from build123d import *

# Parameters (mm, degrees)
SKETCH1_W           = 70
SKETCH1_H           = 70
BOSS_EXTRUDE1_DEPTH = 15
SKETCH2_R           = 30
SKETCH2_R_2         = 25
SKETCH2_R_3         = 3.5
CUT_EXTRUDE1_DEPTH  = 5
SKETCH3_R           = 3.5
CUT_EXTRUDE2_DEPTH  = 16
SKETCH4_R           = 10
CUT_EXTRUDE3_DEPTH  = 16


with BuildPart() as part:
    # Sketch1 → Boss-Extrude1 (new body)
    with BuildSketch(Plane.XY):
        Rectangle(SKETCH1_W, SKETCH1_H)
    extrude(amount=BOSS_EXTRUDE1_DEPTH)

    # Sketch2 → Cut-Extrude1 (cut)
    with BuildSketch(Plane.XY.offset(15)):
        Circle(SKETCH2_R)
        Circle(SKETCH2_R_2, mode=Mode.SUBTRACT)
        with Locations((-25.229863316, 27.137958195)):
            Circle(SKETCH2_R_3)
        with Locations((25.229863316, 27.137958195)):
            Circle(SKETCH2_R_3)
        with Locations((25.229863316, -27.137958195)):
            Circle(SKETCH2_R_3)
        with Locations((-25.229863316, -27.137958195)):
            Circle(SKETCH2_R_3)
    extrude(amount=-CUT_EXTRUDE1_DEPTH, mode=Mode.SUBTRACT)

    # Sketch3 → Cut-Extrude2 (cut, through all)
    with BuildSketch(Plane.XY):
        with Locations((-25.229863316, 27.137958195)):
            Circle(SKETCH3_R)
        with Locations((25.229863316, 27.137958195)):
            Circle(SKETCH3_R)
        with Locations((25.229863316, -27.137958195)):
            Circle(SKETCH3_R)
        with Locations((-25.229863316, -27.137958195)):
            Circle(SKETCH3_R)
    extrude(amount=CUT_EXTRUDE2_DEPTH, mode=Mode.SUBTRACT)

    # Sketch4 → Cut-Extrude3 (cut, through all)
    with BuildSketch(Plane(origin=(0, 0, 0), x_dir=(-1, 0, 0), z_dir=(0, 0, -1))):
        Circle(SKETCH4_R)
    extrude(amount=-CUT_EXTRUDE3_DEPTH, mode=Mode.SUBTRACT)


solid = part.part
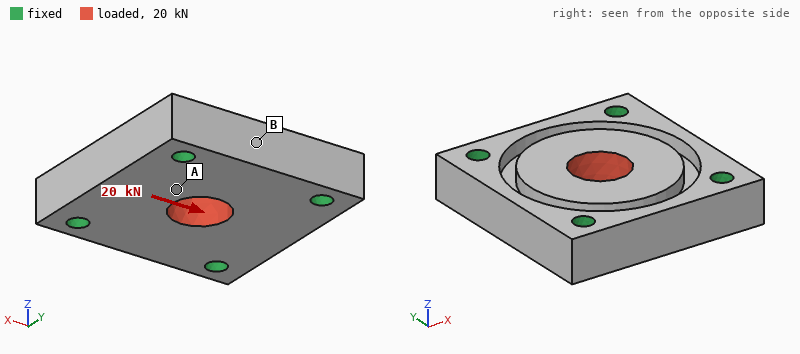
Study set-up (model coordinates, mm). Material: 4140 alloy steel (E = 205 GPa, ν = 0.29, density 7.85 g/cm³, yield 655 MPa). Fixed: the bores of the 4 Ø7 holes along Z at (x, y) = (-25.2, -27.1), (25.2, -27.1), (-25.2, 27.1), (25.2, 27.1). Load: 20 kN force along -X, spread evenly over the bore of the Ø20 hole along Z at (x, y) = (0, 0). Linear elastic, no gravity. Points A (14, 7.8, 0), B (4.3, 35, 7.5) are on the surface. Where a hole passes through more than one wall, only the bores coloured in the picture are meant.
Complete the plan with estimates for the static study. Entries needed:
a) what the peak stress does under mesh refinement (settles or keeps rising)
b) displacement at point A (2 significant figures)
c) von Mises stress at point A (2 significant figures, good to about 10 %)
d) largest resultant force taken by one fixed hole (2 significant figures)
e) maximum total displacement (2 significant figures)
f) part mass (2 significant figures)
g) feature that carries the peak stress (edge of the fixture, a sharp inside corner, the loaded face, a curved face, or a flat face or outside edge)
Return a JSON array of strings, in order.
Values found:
["keeps rising", "3.4 µm", "19 MPa", "5.4 kN", "5.1 µm", "490 g", "edge of the fixture"]
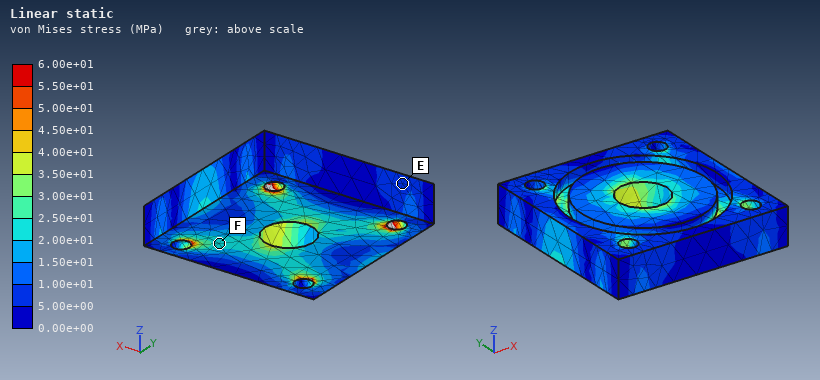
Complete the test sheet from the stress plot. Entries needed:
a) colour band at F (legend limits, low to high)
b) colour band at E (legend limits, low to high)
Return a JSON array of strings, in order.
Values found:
["2.00e+01 to 2.50e+01 MPa", "5.00e+00 to 1.00e+01 MPa"]
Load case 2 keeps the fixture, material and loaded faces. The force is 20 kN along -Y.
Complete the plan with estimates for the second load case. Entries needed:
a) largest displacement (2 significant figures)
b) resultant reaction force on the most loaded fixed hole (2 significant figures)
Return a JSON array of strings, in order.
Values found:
["4.7 µm", "5.4 kN"]
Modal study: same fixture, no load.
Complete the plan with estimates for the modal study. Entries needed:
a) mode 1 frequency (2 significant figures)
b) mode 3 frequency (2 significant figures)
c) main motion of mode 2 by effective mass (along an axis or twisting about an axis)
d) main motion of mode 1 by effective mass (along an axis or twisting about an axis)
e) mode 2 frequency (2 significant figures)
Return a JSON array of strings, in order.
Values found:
["15 kHz", "22 kHz", "twisting about Y", "along Z", "20 kHz"]
